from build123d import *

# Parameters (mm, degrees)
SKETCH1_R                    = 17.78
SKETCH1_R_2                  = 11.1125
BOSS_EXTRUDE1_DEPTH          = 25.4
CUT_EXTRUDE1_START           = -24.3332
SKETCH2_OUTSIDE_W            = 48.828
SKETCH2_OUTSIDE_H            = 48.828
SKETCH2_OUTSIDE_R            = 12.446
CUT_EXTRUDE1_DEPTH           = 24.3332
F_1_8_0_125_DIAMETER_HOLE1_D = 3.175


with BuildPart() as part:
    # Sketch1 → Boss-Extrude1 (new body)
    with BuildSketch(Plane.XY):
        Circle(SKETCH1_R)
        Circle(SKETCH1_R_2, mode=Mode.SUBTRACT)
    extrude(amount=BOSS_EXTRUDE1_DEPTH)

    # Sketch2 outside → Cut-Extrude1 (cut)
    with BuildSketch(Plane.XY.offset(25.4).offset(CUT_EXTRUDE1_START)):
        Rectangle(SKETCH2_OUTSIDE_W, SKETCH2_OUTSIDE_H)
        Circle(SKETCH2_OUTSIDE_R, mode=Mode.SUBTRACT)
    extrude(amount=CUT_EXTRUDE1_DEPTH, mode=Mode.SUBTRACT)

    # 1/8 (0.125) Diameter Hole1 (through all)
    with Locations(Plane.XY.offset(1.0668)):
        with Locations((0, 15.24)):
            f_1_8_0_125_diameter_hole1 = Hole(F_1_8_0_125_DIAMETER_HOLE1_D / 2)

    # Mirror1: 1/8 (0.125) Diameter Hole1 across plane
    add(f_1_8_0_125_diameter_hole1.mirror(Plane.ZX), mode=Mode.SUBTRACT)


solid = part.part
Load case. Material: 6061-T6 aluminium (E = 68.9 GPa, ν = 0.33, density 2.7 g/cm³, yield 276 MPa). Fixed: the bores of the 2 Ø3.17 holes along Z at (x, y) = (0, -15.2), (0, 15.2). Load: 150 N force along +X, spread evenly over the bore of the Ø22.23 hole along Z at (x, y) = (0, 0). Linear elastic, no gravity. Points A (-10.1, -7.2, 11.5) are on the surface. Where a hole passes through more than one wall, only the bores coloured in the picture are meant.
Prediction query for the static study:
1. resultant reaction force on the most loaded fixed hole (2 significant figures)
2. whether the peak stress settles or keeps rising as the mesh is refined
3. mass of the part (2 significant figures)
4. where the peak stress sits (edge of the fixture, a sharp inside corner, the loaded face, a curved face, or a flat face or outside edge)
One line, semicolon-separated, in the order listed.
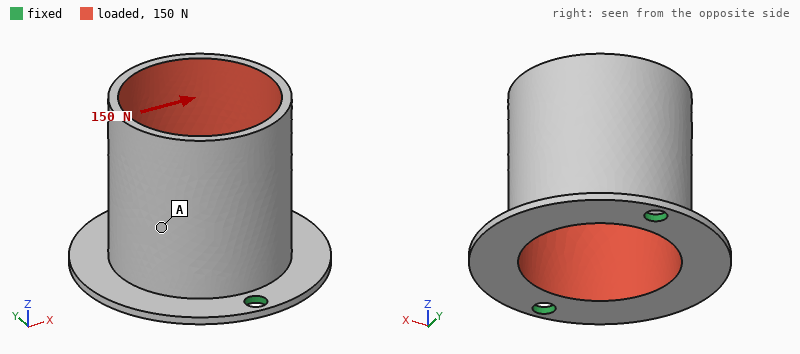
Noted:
75 N; keeps rising; 8.2 g; edge of the fixture
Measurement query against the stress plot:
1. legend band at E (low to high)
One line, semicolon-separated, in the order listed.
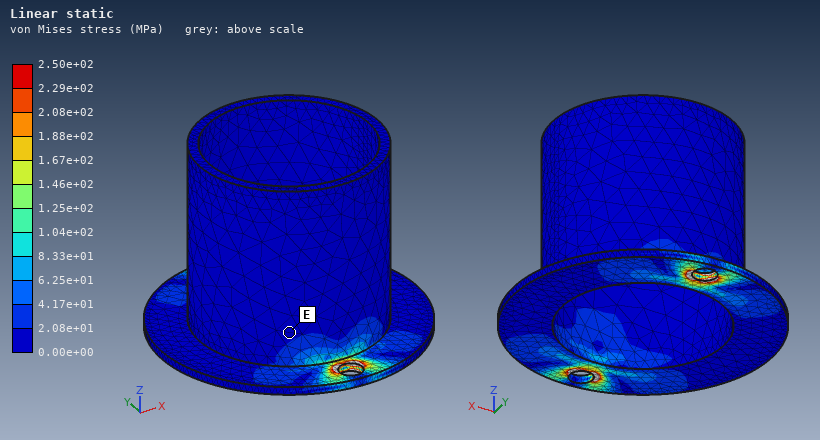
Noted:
0.00e+00 to 2.08e+01 MPa
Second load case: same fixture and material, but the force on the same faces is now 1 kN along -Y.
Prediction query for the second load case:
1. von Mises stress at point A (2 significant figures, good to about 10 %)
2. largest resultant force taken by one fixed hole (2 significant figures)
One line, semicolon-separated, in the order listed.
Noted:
23 MPa; 680 N
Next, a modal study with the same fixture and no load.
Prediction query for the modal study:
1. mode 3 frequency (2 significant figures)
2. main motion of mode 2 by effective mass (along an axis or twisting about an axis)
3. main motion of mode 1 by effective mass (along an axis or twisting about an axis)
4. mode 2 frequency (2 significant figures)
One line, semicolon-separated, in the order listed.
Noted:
6900 Hz; along Z; along X; 6200 Hz
